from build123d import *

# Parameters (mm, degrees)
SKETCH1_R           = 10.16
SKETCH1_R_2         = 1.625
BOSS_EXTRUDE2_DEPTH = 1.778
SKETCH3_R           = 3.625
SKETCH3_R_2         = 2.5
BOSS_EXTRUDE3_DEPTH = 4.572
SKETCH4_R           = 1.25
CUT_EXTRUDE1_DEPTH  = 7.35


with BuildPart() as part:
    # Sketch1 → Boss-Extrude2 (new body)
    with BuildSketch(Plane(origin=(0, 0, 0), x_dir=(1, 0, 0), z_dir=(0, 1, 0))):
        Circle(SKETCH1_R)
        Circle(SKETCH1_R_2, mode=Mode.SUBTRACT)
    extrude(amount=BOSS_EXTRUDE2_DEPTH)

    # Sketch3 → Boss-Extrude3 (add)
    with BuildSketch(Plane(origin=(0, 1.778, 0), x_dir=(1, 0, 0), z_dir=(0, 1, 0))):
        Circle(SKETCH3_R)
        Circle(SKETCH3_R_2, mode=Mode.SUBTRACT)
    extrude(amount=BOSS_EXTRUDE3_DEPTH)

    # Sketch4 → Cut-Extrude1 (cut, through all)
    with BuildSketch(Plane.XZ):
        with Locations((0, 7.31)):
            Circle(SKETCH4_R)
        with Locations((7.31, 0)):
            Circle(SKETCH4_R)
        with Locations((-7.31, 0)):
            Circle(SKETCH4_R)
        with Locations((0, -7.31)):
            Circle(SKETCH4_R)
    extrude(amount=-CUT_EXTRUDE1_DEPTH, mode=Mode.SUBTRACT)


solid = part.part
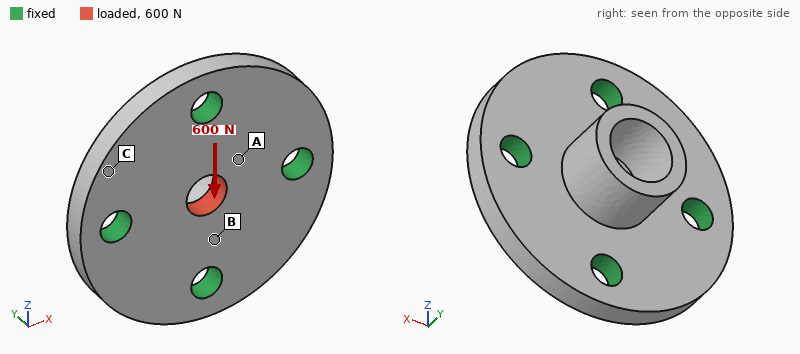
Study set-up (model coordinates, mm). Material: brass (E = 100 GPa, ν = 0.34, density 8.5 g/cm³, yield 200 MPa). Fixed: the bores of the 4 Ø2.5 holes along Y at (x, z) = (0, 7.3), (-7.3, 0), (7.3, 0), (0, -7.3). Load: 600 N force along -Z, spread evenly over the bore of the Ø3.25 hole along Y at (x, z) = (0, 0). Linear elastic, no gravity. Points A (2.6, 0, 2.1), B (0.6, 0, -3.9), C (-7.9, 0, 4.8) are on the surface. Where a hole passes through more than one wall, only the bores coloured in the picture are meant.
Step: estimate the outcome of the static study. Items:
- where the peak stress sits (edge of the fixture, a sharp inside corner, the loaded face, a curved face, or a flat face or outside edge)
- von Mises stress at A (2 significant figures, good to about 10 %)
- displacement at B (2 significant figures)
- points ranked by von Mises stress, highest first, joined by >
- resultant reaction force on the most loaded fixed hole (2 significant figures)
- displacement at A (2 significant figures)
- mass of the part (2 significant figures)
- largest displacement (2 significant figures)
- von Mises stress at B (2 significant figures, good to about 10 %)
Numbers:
the loaded face
17 MPa
0.69 µm
B > A > C
210 N
0.86 µm
5.3 g
1.5 µm
31 MPa
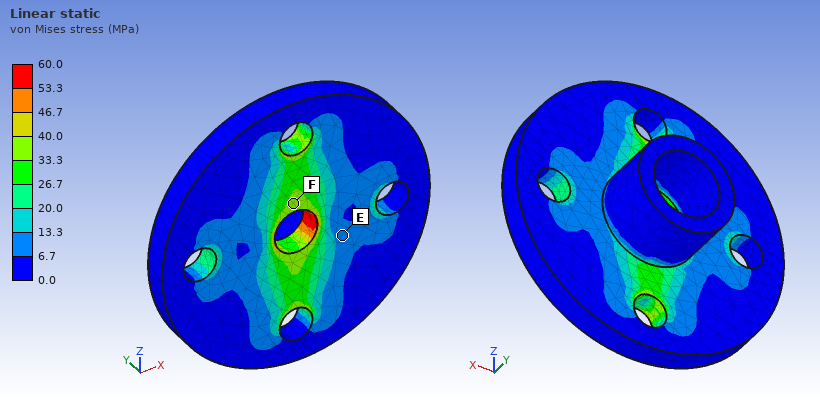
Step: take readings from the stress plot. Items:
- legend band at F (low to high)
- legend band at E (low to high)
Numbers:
33.3 to 40.0 MPa
6.7 to 13.3 MPa
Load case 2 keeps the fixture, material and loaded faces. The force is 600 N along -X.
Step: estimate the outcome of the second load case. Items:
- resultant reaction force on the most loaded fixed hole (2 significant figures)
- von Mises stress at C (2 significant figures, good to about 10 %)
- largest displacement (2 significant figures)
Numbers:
210 N
4.8 MPa
1.5 µm
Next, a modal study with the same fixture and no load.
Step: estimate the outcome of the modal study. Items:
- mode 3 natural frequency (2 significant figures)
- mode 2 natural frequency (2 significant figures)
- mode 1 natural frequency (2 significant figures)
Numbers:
42 kHz
42 kHz
42 kHz
